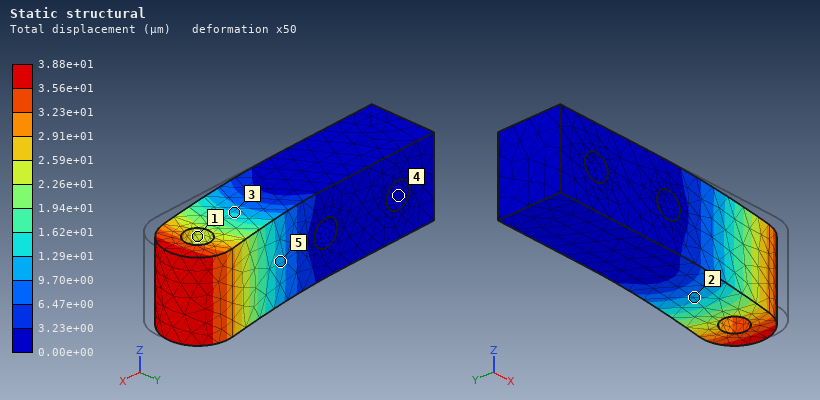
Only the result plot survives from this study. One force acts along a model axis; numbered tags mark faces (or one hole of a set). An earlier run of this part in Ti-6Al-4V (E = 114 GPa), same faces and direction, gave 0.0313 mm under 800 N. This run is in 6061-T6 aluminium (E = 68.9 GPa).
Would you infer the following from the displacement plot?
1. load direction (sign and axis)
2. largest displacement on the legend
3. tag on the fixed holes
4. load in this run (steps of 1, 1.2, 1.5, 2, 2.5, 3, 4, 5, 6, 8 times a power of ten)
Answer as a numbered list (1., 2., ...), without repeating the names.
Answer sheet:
1. +Y
2. 3.88e+01 µm
3. 4
4. 600 N
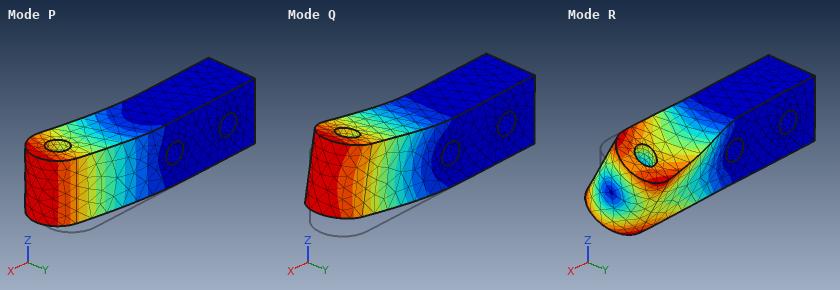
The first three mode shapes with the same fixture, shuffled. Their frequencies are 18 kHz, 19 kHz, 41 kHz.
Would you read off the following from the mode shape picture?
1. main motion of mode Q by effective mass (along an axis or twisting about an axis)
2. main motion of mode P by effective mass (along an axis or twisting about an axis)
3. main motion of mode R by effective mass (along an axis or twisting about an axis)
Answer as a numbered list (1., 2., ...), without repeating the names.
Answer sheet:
1. along Z
2. along Y
3. twisting about X
